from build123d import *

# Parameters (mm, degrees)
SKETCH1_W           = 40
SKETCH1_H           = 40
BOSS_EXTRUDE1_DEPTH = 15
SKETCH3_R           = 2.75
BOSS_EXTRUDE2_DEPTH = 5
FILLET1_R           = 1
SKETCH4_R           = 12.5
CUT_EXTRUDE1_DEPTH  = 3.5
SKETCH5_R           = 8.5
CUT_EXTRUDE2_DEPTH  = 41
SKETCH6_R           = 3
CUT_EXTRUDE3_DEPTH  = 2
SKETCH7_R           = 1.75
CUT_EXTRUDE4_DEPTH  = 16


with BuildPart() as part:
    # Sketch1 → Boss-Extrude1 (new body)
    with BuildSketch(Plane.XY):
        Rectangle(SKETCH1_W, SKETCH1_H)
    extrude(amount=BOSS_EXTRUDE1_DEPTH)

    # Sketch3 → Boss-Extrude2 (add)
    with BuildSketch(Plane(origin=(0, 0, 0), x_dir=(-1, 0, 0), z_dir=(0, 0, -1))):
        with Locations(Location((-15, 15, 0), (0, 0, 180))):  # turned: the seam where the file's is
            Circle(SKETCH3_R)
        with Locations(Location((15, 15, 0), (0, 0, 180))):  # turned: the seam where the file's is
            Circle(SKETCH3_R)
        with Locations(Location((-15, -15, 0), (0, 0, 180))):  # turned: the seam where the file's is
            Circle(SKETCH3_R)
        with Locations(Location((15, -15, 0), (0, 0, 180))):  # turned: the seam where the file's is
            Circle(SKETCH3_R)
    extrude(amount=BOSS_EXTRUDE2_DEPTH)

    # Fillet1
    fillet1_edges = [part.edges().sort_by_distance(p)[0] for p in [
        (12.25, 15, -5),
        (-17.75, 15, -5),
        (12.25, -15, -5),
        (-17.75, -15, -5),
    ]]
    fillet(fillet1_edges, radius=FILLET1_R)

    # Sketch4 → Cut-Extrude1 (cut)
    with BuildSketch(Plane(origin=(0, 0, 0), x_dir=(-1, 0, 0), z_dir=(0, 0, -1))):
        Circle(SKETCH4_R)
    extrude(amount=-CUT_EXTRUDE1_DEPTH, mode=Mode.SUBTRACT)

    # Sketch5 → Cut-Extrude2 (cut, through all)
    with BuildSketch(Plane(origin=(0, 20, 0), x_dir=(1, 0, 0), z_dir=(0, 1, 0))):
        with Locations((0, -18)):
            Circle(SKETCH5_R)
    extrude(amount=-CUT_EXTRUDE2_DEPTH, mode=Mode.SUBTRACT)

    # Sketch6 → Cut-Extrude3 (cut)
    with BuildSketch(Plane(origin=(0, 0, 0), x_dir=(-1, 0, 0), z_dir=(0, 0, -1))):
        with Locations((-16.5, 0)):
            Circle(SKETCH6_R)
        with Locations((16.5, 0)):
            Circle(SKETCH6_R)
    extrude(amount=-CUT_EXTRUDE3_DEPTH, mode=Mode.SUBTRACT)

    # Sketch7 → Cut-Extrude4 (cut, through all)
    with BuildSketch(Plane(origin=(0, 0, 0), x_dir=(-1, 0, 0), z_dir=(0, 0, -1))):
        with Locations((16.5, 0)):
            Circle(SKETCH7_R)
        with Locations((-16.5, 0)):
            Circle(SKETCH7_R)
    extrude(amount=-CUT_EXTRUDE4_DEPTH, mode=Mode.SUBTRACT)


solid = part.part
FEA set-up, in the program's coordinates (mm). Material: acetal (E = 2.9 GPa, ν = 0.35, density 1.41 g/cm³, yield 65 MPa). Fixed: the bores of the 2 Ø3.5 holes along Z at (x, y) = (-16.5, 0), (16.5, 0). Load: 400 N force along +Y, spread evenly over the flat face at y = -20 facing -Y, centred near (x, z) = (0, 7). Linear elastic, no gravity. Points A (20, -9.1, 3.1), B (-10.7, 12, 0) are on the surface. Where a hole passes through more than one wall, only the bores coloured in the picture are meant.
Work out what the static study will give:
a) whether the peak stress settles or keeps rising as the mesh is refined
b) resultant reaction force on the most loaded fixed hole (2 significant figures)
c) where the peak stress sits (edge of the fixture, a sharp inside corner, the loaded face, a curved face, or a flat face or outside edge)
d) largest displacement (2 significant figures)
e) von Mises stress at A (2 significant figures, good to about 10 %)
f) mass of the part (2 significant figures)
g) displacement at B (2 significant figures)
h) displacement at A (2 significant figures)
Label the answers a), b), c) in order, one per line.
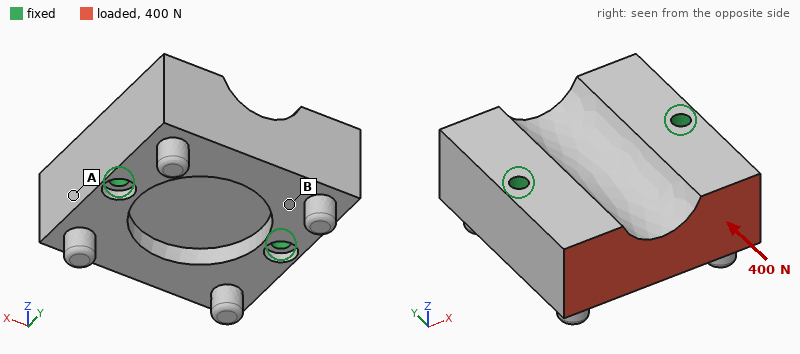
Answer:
a) keeps rising
b) 200 N
c) edge of the fixture
d) 17 µm
e) 1.0 MPa
f) 28 g
g) 3.3 µm
h) 5.2 µm
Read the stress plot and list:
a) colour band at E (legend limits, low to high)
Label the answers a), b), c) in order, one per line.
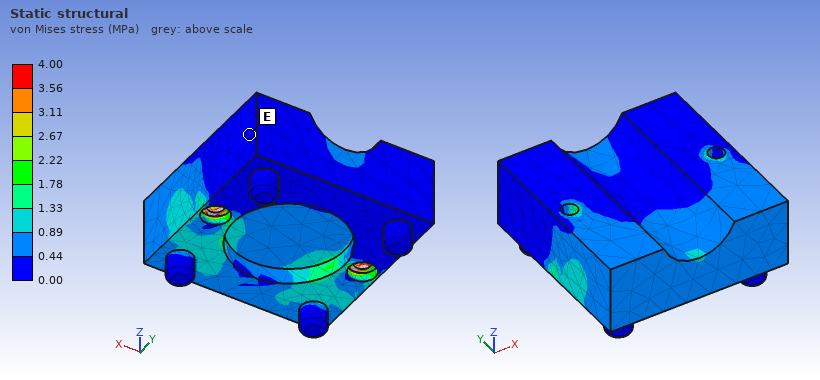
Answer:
a) 0.00 to 0.44 MPa
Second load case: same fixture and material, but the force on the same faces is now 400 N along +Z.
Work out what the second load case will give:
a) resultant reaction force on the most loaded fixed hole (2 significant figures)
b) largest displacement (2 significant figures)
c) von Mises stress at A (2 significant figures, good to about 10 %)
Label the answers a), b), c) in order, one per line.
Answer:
a) 200 N
b) 0.12 mm
c) 3.1 MPa
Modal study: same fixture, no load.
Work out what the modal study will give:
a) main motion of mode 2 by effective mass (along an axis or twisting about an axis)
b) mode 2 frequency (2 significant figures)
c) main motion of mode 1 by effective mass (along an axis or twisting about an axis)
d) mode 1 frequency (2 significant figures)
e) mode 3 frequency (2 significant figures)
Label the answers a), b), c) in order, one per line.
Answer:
a) along Z
b) 4800 Hz
c) twisting about X
d) 4000 Hz
e) 5900 Hz
